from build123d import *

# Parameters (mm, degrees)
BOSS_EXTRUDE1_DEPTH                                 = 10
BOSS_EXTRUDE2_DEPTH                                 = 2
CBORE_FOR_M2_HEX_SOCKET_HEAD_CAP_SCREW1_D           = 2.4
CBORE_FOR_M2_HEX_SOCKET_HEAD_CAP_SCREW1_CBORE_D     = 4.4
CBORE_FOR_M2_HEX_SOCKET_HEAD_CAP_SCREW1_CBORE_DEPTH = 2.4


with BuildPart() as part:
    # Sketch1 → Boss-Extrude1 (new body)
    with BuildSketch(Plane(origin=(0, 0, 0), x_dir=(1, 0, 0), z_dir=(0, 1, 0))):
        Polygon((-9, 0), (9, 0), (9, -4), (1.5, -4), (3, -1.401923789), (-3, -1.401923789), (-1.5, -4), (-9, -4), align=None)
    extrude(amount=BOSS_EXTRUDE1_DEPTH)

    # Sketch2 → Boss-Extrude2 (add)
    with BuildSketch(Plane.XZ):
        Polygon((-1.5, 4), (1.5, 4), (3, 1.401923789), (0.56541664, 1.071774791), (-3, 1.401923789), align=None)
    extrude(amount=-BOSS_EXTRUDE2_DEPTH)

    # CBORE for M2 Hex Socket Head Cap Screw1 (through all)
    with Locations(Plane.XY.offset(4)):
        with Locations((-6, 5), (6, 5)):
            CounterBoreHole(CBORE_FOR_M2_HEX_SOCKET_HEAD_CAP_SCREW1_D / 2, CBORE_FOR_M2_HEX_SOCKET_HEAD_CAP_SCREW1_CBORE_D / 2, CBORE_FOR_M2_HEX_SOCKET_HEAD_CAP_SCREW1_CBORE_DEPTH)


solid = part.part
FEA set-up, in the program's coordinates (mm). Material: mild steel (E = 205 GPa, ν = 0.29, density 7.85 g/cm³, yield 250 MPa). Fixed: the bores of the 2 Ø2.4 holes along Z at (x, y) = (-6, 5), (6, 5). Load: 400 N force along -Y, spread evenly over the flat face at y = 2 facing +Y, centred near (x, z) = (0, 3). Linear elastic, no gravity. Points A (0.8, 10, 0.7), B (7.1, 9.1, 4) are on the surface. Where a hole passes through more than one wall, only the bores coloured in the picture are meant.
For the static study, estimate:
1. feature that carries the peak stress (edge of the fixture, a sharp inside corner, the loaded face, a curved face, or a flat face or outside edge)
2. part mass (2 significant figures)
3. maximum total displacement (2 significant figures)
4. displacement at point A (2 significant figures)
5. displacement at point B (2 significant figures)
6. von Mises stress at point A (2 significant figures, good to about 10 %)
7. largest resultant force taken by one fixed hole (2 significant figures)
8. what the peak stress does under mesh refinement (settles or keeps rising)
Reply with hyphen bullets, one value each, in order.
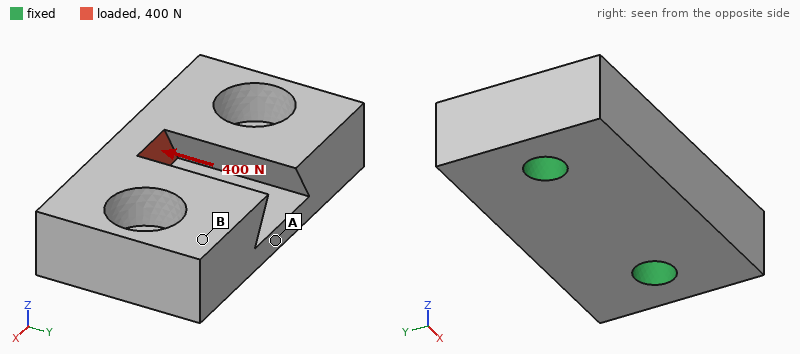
- edge of the fixture
- 4.2 g
- 4.4 µm
- 1.4 µm
- 1.6 µm
- 21 MPa
- 210 N
- keeps rising
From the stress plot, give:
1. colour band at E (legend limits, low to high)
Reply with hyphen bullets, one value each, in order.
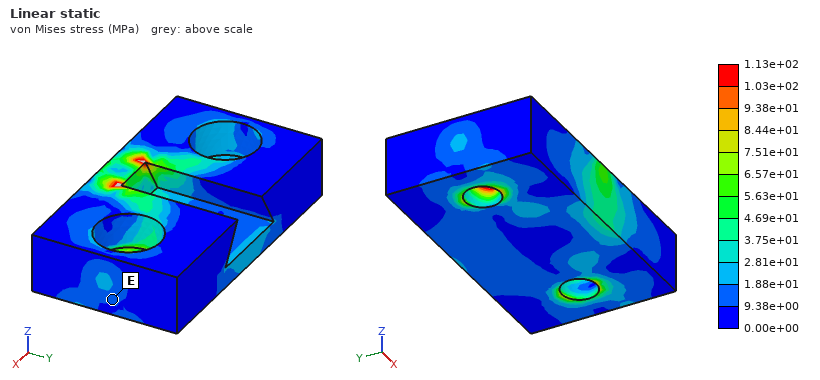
- 9.38e+00 to 1.88e+01 MPa
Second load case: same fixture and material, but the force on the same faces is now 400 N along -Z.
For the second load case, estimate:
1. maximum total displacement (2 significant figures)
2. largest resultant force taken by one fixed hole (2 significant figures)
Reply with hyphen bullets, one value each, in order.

- 5.7 µm
- 210 N
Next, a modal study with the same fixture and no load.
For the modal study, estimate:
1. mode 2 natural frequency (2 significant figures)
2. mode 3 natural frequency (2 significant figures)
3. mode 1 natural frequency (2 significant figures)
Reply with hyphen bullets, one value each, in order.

- 48 kHz
- 49 kHz
- 35 kHz
